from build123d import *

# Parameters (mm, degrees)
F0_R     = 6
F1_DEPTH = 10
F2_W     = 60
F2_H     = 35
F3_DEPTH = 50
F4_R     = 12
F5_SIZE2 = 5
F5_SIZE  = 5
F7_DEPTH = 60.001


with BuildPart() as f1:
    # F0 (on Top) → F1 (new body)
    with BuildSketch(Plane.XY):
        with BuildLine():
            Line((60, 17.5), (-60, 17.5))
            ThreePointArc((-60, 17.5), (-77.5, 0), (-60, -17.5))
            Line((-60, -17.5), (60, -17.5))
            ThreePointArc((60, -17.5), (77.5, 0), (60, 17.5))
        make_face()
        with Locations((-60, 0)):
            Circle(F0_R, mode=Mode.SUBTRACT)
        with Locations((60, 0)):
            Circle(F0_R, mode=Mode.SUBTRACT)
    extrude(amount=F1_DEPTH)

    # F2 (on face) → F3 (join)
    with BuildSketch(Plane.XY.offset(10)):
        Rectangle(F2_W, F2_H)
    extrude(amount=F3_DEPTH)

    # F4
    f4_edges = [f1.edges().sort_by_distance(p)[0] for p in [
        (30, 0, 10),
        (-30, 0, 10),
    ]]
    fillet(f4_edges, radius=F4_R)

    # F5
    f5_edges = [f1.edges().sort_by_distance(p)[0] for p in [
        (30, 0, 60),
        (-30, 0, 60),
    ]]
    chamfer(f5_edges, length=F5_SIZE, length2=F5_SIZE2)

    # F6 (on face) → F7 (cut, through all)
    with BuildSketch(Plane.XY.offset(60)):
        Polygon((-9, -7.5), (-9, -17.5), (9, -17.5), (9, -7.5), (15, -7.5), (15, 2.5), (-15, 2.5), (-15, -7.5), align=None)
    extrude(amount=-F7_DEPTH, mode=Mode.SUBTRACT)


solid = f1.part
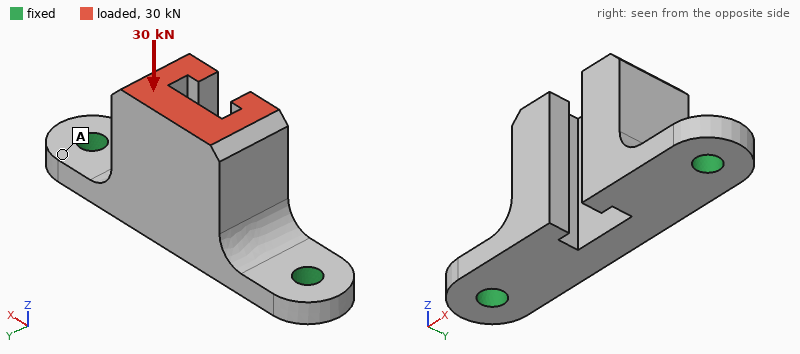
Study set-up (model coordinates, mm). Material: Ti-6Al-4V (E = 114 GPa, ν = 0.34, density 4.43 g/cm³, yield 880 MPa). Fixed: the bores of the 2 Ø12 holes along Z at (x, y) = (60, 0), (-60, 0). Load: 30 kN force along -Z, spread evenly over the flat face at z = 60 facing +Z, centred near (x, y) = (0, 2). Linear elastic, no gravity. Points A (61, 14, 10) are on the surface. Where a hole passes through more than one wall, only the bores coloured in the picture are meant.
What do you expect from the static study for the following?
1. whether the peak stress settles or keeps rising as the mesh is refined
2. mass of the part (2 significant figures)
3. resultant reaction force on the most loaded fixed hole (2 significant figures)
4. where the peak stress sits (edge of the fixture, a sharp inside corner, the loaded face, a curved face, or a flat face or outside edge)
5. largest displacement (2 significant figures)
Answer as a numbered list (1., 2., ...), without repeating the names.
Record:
1. keeps rising
2. 560 g
3. 18 kN
4. edge of the fixture
5. 0.18 mm
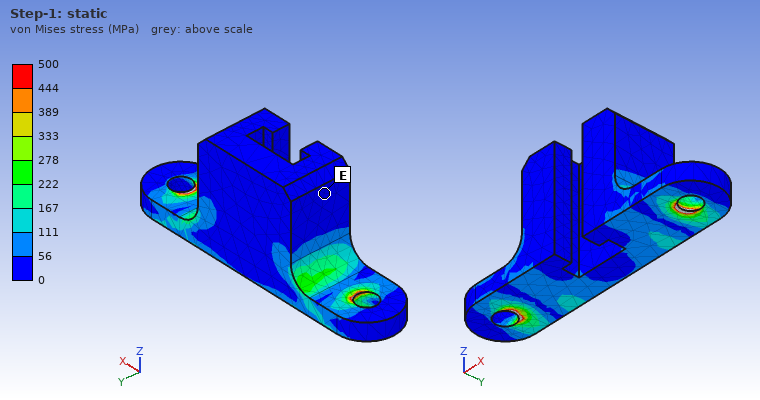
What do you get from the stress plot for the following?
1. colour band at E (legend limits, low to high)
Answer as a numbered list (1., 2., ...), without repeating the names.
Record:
1. 0 to 56 MPa
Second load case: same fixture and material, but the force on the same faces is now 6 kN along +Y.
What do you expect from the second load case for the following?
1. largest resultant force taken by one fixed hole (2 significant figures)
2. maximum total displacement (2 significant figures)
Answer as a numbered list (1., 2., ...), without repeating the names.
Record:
1. 3.6 kN
2. 0.48 mm
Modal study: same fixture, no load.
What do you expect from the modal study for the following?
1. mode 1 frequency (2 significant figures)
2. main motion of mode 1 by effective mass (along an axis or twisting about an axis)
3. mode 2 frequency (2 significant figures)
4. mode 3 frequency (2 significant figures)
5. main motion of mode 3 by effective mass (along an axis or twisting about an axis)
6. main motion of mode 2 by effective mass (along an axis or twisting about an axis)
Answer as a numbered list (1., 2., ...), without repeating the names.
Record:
1. 1500 Hz
2. along Y
3. 3700 Hz
4. 4600 Hz
5. along X
6. along Z
